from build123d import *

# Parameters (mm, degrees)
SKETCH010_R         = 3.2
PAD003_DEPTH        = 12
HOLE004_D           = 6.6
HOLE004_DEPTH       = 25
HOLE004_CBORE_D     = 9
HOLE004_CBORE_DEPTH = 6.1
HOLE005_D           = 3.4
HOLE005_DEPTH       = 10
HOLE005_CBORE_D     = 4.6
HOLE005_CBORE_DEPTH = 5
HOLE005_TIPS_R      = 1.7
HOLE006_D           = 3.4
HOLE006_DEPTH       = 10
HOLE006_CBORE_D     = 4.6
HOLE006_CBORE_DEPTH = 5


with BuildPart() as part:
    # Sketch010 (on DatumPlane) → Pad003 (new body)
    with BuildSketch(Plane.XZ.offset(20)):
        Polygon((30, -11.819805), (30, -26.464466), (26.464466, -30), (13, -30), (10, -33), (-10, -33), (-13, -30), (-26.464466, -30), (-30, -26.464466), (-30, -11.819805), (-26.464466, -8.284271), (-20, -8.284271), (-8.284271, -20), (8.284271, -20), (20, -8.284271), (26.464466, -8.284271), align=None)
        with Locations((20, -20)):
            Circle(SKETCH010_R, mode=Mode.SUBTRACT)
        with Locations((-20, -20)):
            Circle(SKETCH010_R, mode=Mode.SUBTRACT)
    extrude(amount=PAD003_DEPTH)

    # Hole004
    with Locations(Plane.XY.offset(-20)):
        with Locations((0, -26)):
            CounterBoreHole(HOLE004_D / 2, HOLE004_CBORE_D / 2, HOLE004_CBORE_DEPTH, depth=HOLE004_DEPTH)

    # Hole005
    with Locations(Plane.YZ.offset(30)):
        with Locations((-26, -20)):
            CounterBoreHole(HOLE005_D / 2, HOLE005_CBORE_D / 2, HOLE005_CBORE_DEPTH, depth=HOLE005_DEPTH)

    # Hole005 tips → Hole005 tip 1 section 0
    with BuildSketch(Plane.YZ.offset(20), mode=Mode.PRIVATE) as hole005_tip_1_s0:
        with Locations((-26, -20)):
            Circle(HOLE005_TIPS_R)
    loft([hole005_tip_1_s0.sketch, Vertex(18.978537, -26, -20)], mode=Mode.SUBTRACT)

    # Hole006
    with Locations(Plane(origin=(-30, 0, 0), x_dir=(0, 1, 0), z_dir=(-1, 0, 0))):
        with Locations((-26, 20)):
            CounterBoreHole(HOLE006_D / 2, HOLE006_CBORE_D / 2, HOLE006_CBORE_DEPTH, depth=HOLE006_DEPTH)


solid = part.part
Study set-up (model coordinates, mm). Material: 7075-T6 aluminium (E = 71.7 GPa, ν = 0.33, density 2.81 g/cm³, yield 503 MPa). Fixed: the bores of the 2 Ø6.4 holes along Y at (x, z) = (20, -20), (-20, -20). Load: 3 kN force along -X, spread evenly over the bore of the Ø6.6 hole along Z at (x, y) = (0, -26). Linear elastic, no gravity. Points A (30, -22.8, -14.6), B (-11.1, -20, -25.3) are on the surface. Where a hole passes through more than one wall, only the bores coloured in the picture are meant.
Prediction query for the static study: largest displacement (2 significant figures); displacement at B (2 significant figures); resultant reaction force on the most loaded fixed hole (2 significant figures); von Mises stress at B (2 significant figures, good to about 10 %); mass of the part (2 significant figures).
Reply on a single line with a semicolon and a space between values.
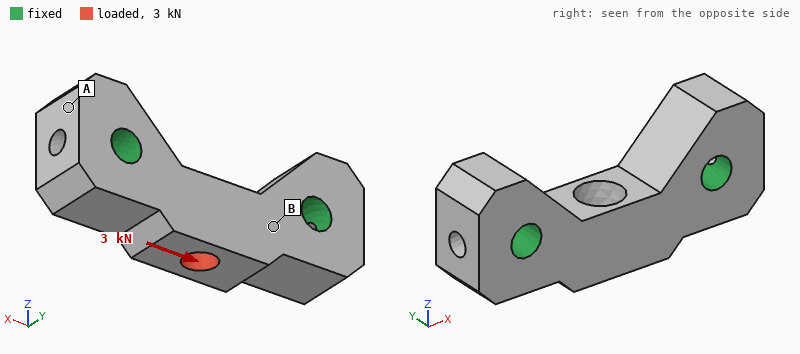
5.1 µm; 1.8 µm; 1.6 kN; 12 MPa; 30 g
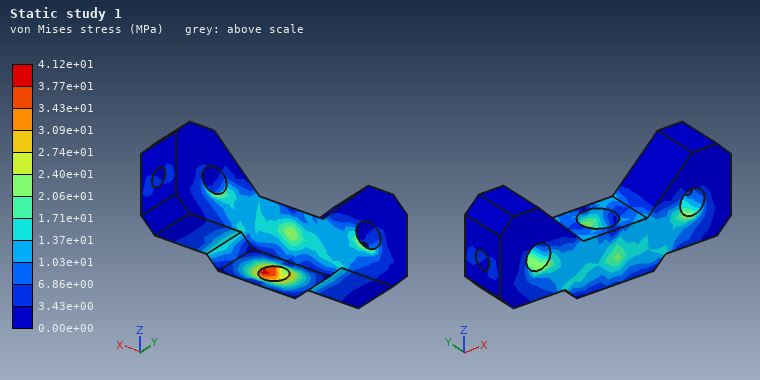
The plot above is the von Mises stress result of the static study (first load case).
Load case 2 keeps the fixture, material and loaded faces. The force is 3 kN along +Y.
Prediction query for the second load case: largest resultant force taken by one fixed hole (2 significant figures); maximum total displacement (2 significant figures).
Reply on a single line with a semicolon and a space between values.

1.5 kN; 28 µm
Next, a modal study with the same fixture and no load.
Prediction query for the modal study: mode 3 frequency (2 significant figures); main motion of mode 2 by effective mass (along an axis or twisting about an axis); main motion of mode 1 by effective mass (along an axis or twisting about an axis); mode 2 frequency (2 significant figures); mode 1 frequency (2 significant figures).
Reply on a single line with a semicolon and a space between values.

42 kHz; along Z; along Y; 32 kHz; 27 kHz
